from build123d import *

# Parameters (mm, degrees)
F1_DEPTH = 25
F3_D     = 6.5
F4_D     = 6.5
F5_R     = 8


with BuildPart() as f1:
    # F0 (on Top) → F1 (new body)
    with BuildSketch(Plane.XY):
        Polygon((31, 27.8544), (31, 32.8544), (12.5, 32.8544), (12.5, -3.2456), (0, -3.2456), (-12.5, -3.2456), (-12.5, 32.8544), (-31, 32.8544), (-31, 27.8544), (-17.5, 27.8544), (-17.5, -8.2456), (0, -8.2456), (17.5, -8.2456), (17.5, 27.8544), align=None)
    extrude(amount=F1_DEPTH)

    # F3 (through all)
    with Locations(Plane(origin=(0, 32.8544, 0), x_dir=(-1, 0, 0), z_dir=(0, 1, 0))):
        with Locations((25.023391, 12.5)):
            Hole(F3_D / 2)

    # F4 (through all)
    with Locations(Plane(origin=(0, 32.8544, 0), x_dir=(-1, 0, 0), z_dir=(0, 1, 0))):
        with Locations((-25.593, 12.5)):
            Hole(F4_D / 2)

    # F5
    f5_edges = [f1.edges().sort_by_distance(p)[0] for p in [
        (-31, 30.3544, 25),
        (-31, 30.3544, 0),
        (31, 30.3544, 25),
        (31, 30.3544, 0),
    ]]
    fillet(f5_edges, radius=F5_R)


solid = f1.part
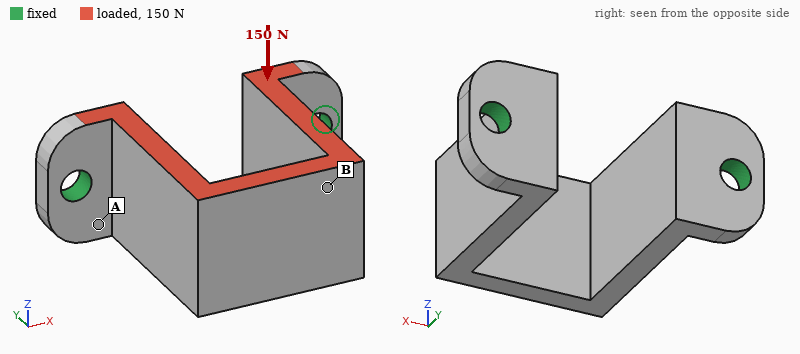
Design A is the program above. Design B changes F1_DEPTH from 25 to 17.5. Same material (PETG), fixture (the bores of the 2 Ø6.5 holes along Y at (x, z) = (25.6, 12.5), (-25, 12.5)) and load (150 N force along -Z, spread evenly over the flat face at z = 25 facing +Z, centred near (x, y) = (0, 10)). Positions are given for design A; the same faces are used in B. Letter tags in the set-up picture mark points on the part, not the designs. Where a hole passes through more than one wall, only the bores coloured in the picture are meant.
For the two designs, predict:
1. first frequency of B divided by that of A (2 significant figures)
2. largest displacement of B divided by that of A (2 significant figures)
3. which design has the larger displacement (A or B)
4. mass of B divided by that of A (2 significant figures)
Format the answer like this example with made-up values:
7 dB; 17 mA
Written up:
0.95; 1.6; B; 0.69
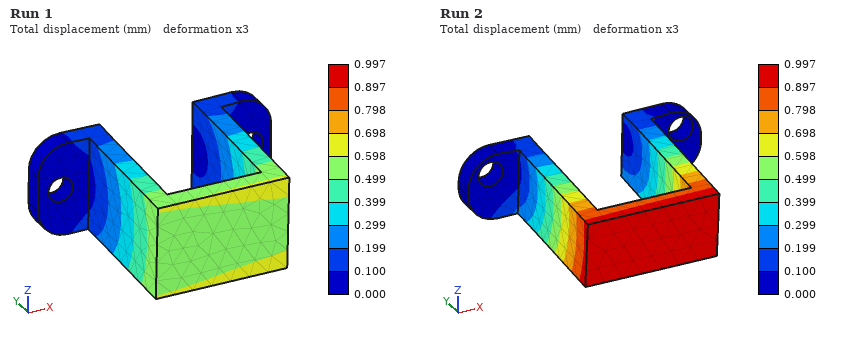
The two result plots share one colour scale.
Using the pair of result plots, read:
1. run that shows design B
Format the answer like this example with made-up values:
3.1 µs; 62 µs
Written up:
Run 2
